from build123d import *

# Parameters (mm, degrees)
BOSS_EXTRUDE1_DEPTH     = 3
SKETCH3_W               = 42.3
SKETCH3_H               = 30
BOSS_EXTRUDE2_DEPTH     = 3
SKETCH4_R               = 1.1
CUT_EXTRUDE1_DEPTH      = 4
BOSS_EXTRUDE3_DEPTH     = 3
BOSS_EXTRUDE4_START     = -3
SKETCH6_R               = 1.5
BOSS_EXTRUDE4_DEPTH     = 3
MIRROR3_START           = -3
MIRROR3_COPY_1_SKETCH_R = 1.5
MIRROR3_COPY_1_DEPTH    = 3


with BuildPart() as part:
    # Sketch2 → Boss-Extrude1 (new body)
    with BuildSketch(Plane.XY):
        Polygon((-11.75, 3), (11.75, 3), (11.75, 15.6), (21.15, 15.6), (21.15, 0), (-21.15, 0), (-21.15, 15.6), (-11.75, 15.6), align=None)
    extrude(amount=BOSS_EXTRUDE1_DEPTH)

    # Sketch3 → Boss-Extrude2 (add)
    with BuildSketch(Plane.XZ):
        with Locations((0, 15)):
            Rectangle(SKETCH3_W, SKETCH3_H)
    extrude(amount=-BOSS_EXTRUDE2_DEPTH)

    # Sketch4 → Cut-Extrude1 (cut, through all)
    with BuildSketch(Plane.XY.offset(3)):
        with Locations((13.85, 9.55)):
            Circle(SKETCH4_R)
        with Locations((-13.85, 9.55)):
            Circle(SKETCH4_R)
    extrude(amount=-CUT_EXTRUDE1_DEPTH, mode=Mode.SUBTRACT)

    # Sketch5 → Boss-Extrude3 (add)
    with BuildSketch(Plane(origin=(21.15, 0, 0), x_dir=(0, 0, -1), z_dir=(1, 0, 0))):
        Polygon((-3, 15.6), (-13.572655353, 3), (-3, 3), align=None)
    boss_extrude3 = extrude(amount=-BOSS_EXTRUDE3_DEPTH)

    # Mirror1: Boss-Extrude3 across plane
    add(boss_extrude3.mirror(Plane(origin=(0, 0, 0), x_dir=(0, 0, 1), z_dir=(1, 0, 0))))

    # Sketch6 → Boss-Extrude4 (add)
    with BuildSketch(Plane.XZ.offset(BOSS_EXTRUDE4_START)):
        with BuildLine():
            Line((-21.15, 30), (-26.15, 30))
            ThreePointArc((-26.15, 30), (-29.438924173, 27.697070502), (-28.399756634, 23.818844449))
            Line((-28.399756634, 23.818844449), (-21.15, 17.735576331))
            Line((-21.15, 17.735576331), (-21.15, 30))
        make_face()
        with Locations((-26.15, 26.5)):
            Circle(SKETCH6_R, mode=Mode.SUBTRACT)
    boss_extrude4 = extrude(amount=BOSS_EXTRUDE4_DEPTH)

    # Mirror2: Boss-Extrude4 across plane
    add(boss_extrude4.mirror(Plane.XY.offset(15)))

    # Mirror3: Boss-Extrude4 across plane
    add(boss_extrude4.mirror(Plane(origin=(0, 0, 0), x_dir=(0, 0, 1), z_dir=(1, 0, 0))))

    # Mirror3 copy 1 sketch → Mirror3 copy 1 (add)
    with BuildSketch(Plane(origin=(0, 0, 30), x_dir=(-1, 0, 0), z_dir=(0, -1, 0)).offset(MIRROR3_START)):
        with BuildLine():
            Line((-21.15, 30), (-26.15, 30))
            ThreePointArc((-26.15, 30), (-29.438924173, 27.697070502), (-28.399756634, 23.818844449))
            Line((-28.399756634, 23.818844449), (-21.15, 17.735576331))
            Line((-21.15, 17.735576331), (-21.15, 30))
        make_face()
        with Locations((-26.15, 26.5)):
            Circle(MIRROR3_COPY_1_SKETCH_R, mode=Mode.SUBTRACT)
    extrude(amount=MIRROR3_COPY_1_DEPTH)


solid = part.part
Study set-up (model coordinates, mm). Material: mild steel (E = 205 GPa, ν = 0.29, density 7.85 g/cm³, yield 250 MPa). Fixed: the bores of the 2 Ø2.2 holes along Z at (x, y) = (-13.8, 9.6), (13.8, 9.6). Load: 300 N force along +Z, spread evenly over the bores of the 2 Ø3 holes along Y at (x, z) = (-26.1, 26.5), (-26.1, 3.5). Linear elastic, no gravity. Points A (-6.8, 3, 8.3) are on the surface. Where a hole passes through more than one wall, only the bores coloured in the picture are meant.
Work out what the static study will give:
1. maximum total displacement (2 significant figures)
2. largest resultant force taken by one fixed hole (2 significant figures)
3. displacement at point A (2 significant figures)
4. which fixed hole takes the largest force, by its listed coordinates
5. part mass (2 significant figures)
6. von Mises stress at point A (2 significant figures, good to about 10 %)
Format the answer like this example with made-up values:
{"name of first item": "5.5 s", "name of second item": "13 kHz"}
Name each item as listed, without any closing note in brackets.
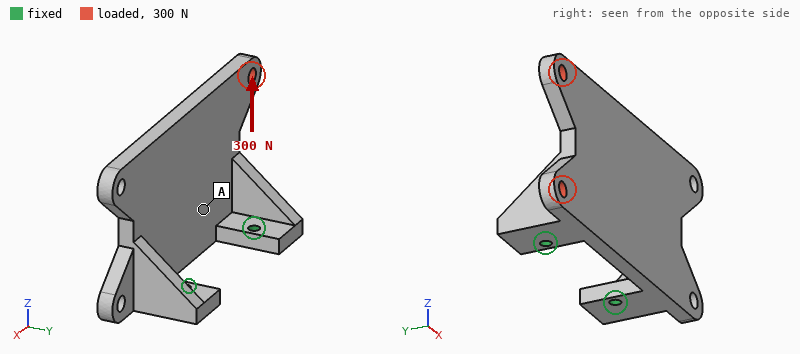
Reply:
{"maximum total displacement": "43 µm", "largest resultant force taken by one fixed hole": "380 N", "displacement at point A": "9.8 µm", "which fixed hole takes the largest force, by its listed coordinates": "(-13.8, 9.6)", "part mass": "44 g", "von Mises stress at point A": "17 MPa"}
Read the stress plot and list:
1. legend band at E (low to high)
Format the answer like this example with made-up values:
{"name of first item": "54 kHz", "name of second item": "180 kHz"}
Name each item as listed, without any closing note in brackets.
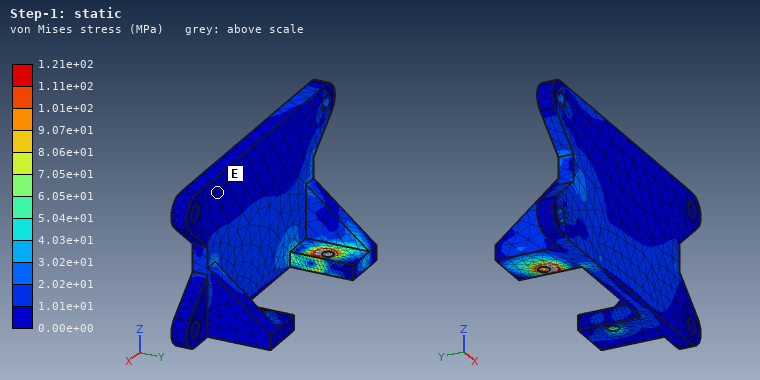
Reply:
{"legend band at E": "0.00e+00 to 1.01e+01 MPa"}
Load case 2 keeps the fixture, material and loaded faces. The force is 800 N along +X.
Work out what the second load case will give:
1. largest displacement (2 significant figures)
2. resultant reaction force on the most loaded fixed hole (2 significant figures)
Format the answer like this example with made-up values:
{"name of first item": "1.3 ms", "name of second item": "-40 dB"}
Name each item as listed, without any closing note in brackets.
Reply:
{"largest displacement": "32 µm", "resultant reaction force on the most loaded fixed hole": "540 N"}
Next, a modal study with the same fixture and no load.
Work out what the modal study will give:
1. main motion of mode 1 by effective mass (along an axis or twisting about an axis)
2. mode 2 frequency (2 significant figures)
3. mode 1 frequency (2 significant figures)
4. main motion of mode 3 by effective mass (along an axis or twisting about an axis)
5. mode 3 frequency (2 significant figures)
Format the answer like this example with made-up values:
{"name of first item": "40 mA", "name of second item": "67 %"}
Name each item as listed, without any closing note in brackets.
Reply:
{"main motion of mode 1 by effective mass": "along Y", "mode 2 frequency": "3800 Hz", "mode 1 frequency": "2200 Hz", "main motion of mode 3 by effective mass": "along X", "mode 3 frequency": "6100 Hz"}
